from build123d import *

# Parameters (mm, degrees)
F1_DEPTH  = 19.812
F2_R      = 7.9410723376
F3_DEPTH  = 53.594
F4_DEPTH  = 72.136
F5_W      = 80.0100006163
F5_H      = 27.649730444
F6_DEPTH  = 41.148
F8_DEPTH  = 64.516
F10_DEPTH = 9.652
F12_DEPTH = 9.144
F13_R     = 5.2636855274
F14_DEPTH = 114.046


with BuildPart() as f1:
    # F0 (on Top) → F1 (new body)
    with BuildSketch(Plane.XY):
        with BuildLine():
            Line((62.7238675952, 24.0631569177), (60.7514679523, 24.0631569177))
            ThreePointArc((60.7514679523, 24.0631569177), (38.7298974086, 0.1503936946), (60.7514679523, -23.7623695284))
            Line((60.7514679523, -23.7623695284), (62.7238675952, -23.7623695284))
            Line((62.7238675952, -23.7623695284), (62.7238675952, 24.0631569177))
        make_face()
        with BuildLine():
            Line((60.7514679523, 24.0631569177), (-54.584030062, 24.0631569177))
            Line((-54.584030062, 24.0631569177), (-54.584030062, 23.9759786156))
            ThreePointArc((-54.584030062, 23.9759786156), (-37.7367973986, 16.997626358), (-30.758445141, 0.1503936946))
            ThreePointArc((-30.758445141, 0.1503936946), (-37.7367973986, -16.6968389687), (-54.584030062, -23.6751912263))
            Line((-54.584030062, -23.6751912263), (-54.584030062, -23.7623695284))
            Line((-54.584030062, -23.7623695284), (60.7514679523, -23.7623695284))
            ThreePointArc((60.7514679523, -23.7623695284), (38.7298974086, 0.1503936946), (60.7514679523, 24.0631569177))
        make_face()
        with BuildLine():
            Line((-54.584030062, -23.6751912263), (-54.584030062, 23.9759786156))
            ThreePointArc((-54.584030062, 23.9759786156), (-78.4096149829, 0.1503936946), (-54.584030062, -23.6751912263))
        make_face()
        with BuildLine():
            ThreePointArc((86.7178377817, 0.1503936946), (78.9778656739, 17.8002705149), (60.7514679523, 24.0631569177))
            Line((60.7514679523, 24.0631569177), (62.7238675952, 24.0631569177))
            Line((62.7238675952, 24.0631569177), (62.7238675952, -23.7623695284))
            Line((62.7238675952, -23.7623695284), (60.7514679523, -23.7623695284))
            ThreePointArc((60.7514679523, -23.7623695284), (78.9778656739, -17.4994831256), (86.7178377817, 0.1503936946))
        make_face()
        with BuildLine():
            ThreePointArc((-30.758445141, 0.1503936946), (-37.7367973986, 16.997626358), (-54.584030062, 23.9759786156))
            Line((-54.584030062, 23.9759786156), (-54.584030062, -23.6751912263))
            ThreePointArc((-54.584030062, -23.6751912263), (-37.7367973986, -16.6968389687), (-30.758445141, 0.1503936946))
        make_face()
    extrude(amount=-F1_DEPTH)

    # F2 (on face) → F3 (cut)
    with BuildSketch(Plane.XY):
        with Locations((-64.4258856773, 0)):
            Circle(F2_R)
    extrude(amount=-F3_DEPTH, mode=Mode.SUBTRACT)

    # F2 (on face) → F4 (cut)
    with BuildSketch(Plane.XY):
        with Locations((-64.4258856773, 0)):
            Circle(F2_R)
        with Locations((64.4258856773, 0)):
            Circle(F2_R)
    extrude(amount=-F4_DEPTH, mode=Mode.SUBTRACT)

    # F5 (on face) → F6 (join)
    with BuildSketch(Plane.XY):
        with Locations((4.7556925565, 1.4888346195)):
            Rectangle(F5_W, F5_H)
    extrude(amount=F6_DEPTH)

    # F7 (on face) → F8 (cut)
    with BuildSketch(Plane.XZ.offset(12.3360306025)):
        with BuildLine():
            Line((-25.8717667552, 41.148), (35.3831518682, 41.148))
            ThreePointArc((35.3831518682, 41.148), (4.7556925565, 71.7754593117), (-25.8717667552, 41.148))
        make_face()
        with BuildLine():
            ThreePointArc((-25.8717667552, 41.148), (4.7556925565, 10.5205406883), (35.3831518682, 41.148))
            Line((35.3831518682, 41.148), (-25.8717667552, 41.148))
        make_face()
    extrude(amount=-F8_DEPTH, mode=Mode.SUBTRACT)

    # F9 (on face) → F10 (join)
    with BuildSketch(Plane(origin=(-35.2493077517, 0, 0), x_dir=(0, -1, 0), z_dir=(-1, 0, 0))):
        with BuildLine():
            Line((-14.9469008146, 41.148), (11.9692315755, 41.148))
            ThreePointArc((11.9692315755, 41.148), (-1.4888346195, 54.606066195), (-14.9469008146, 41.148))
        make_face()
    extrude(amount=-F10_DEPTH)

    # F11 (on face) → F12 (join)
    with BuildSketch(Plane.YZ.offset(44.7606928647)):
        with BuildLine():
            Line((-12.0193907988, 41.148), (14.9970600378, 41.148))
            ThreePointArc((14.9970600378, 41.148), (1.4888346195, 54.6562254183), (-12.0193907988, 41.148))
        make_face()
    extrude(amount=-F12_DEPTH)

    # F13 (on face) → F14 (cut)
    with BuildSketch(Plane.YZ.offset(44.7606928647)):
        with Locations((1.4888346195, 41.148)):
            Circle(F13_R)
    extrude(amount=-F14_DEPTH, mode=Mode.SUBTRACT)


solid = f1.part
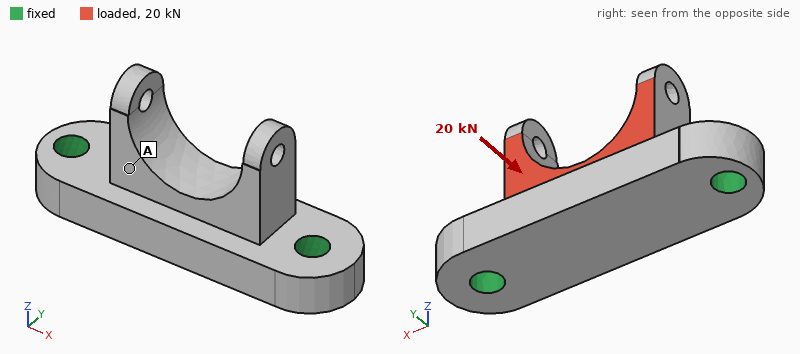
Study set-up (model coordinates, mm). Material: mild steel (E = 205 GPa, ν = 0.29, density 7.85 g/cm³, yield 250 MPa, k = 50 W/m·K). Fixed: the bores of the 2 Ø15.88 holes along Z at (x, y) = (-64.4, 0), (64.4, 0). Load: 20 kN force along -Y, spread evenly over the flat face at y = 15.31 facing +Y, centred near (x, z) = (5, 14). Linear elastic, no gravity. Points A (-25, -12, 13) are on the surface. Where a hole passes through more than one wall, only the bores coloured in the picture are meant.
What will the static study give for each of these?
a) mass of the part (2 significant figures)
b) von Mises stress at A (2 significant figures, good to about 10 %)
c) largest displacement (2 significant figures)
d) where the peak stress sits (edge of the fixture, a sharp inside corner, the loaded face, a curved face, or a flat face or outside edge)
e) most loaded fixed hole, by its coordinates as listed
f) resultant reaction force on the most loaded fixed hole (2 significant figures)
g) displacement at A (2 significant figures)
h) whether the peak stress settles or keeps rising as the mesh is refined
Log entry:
1.5 kg
22 MPa
81 µm
edge of the fixture
(64.4, 0)
11 kN
34 µm
keeps rising
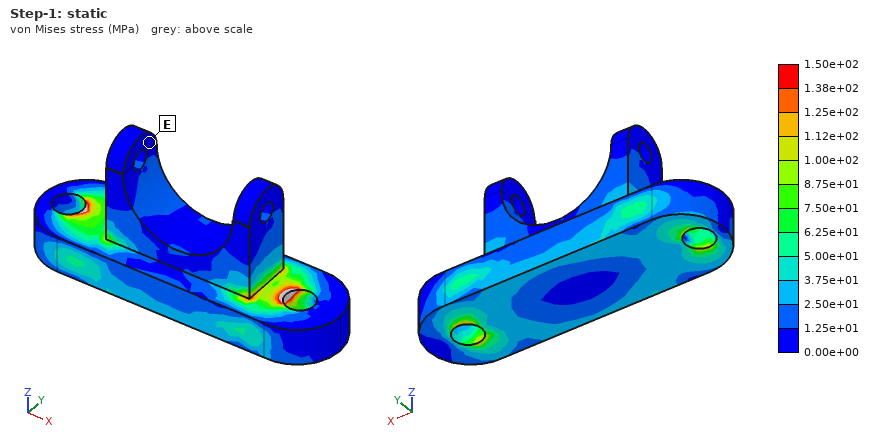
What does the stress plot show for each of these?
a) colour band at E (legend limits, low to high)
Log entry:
0.00e+00 to 1.25e+01 MPa
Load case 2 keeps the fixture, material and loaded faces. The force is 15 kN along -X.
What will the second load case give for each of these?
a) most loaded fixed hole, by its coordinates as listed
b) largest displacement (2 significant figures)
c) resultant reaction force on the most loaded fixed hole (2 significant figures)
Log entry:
(64.4, 0)
21 µm
9.0 kN
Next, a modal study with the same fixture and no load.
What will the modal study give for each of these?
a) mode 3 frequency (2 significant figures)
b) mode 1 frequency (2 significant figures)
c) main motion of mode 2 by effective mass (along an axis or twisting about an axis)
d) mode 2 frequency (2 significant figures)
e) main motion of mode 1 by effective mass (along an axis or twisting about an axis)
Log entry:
7300 Hz
4400 Hz
along Z
5500 Hz
along Y
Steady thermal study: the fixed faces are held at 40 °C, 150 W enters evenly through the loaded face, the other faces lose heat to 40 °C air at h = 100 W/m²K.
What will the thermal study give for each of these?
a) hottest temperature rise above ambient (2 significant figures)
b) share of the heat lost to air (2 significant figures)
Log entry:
65 K
46 %
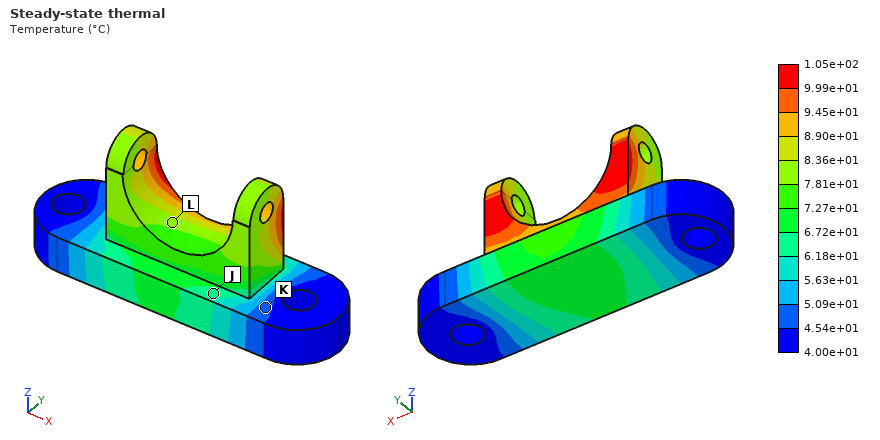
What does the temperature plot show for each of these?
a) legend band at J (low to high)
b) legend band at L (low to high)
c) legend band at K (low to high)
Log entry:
6.18e+01 to 6.72e+01 °C
7.81e+01 to 8.36e+01 °C
4.54e+01 to 5.09e+01 °C
